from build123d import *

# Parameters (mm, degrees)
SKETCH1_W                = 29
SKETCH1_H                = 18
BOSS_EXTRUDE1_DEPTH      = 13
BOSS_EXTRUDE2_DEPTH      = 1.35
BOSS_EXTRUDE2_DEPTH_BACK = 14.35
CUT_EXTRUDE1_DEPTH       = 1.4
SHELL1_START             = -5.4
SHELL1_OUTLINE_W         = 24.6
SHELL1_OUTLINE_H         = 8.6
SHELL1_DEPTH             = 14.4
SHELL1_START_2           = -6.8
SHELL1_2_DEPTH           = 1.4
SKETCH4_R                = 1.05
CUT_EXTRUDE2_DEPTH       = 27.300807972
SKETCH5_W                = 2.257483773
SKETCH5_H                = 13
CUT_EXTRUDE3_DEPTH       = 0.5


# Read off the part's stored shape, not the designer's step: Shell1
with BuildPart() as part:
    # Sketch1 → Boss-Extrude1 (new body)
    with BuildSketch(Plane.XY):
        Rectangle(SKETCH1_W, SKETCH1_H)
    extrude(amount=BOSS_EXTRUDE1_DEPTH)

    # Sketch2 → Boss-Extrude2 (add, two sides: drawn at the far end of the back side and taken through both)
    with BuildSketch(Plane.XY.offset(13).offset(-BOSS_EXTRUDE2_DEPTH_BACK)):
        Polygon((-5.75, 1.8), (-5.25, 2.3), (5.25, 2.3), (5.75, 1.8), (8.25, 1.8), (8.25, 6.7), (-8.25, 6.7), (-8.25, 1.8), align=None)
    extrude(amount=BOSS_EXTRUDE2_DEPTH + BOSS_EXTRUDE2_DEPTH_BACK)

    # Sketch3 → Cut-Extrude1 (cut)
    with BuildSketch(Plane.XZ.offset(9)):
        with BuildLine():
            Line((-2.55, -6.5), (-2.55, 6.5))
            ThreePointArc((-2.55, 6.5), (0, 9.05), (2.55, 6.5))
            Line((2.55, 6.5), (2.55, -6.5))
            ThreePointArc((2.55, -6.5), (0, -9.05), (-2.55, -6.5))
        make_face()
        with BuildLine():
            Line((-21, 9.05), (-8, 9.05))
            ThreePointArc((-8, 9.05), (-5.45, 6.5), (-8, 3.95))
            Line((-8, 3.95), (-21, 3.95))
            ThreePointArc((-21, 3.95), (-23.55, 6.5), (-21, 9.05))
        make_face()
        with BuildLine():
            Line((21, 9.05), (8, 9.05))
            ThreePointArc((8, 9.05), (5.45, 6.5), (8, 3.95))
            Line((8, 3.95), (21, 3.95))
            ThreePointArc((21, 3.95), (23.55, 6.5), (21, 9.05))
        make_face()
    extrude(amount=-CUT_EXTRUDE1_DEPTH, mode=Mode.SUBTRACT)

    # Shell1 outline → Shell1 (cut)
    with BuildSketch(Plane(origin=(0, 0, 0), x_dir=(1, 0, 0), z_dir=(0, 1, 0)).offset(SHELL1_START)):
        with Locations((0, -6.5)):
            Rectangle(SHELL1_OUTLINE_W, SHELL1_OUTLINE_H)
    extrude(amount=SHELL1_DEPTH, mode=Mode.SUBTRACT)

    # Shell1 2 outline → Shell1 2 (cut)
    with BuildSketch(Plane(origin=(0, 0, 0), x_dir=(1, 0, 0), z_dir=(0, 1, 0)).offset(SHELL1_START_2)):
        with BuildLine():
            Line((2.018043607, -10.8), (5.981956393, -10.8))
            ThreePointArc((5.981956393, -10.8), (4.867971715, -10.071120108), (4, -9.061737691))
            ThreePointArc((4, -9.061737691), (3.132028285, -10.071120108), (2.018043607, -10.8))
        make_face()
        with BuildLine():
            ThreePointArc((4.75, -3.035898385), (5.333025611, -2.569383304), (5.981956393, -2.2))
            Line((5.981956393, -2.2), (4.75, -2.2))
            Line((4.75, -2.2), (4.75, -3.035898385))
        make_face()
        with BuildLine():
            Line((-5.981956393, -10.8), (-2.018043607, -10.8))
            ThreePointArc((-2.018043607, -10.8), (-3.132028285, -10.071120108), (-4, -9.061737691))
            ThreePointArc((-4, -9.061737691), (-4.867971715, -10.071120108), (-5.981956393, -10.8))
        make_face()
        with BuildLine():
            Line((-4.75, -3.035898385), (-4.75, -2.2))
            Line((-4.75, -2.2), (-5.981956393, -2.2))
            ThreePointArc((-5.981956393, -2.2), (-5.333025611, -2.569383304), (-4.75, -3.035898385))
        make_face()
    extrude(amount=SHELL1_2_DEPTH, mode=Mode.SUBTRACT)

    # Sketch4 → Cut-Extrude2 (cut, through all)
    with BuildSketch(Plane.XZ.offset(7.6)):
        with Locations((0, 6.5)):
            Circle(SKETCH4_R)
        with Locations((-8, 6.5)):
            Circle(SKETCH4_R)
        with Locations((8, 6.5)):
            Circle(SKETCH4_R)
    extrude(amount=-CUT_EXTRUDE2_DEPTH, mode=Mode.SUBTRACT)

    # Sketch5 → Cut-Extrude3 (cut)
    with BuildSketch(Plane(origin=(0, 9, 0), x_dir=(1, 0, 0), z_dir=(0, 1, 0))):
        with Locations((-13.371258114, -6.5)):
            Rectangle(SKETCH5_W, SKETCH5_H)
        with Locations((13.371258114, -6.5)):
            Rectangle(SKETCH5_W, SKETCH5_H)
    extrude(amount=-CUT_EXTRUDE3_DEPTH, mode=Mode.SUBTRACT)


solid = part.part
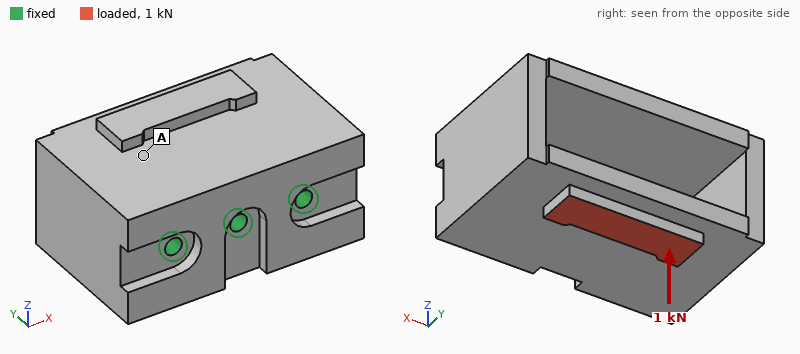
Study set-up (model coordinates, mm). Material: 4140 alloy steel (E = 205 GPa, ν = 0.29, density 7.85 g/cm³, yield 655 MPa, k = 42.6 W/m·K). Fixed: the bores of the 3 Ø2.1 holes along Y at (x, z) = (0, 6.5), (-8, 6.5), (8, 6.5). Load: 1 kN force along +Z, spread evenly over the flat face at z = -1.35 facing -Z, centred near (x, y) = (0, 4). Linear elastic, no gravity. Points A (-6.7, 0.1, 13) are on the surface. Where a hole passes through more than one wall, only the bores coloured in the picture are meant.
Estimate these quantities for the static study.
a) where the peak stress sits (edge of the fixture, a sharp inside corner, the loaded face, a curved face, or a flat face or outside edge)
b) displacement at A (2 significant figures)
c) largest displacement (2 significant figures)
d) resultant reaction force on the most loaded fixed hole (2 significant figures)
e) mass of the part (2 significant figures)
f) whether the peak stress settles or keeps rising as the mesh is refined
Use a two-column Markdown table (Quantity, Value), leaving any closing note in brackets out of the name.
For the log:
| Quantity | Value |
|---|---|
| where the peak stress sits | edge of the fixture |
| displacement at A | 22 µm |
| largest displacement | 78 µm |
| resultant reaction force on the most loaded fixed hole | 550 N |
| mass of the part | 29 g |
| whether the peak stress settles or keeps rising as the mesh is refined | keeps rising |
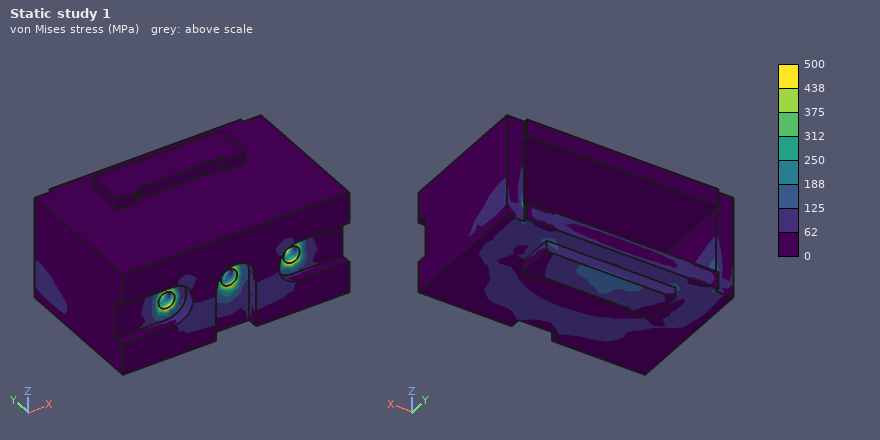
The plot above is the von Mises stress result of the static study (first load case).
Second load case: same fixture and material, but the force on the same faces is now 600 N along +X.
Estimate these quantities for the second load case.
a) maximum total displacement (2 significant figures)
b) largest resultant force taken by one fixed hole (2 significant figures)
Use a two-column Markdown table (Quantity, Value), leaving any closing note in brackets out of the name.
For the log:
| Quantity | Value |
|---|---|
| maximum total displacement | 6.7 µm |
| largest resultant force taken by one fixed hole | 490 N |
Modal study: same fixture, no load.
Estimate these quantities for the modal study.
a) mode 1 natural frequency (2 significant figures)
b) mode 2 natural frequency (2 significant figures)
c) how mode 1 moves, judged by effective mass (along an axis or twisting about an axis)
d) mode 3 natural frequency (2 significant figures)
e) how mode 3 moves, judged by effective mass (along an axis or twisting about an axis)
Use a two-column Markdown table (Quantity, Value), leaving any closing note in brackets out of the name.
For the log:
| Quantity | Value |
|---|---|
| mode 1 natural frequency | 6400 Hz |
| mode 2 natural frequency | 12 kHz |
| how mode 1 moves, judged by effective mass | along Z |
| mode 3 natural frequency | 14 kHz |
| how mode 3 moves, judged by effective mass | along X |
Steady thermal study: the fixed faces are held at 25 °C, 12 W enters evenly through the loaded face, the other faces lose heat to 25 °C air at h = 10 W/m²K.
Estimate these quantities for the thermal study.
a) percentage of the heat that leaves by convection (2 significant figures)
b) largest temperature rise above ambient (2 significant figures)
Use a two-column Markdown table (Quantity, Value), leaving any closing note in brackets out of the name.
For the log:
| Quantity | Value |
|---|---|
| percentage of the heat that leaves by convection | 5.3 % |
| largest temperature rise above ambient | 63 K |
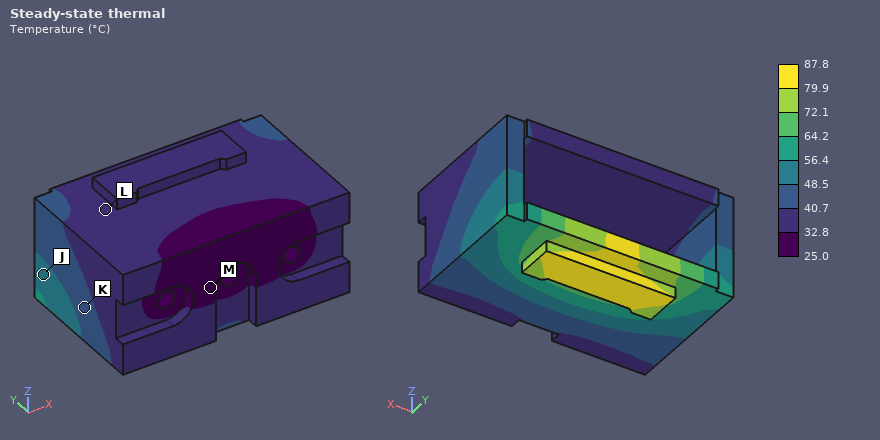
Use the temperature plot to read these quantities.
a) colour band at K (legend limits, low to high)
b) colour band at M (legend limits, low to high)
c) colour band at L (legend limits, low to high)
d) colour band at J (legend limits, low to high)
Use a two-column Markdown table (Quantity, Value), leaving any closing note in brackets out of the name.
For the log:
| Quantity | Value |
|---|---|
| colour band at K | 40.7 to 48.5 °C |
| colour band at M | 25.0 to 32.8 °C |
| colour band at L | 32.8 to 40.7 °C |
| colour band at J | 48.5 to 56.4 °C |
